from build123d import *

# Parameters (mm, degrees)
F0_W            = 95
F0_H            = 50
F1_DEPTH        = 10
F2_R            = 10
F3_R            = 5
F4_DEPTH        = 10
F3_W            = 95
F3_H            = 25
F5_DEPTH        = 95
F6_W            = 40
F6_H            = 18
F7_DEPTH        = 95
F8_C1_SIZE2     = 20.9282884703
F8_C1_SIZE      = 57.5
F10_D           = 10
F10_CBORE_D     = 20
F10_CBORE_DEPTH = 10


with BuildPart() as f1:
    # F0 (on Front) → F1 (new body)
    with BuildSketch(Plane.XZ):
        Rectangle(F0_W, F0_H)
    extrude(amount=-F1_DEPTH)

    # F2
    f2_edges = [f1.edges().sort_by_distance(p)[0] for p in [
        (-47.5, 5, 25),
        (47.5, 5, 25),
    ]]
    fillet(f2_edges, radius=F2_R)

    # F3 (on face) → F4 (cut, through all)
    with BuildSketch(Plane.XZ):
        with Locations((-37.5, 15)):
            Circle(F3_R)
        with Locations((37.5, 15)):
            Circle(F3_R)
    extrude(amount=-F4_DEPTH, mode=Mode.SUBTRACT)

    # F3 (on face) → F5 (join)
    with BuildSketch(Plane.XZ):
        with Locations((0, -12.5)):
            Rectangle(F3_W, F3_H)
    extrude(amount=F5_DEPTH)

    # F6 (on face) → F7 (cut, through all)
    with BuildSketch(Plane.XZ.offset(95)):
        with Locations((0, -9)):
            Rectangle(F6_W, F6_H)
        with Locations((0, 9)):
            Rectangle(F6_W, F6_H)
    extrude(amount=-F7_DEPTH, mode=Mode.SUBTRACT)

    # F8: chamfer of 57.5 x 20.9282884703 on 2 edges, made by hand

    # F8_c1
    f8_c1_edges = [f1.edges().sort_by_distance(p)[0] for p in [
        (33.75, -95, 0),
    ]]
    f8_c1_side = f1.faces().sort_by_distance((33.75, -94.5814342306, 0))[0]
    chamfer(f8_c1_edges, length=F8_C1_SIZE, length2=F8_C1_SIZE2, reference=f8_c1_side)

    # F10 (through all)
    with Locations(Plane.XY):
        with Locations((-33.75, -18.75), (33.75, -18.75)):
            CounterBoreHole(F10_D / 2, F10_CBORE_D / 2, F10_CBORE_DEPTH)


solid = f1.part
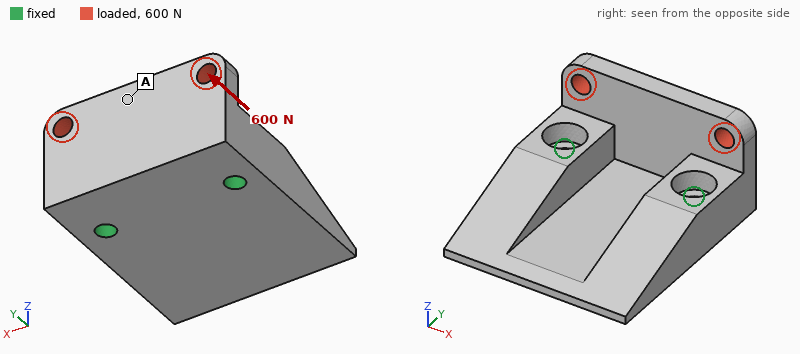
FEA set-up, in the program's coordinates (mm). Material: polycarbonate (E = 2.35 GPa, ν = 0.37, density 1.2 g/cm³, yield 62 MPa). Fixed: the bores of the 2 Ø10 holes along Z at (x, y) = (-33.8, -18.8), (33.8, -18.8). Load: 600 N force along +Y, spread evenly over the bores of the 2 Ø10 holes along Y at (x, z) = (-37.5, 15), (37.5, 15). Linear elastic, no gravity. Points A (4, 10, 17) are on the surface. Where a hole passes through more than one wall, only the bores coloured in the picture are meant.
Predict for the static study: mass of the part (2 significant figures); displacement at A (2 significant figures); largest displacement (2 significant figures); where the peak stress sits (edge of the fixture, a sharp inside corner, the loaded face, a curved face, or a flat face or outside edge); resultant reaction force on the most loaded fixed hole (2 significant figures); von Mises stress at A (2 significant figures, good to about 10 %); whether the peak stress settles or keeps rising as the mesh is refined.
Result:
190 g
0.26 mm
0.45 mm
edge of the fixture
300 N
1.5 MPa
keeps rising
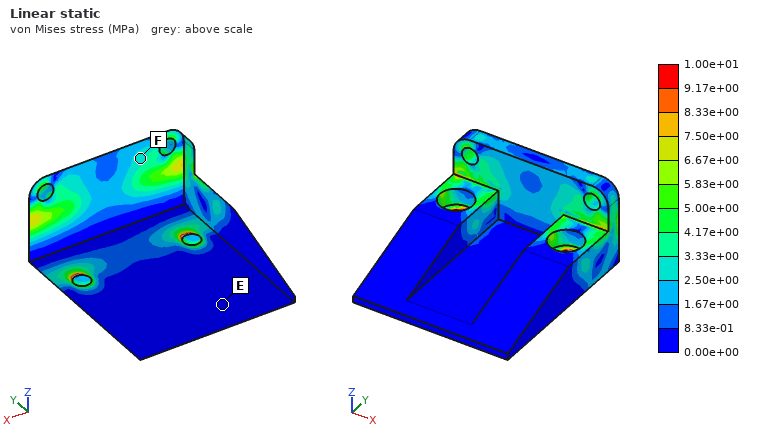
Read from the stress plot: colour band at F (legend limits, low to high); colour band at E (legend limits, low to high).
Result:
2.50e+00 to 3.33e+00 MPa
0.00e+00 to 8.33e-01 MPa
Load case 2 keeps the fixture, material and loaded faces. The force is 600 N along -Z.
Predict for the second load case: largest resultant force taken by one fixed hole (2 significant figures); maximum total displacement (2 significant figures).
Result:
300 N
0.14 mm
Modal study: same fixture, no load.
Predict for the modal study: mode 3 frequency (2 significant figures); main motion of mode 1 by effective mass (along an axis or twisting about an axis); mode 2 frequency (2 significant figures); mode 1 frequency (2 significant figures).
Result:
1400 Hz
along Z
1200 Hz
810 Hz
